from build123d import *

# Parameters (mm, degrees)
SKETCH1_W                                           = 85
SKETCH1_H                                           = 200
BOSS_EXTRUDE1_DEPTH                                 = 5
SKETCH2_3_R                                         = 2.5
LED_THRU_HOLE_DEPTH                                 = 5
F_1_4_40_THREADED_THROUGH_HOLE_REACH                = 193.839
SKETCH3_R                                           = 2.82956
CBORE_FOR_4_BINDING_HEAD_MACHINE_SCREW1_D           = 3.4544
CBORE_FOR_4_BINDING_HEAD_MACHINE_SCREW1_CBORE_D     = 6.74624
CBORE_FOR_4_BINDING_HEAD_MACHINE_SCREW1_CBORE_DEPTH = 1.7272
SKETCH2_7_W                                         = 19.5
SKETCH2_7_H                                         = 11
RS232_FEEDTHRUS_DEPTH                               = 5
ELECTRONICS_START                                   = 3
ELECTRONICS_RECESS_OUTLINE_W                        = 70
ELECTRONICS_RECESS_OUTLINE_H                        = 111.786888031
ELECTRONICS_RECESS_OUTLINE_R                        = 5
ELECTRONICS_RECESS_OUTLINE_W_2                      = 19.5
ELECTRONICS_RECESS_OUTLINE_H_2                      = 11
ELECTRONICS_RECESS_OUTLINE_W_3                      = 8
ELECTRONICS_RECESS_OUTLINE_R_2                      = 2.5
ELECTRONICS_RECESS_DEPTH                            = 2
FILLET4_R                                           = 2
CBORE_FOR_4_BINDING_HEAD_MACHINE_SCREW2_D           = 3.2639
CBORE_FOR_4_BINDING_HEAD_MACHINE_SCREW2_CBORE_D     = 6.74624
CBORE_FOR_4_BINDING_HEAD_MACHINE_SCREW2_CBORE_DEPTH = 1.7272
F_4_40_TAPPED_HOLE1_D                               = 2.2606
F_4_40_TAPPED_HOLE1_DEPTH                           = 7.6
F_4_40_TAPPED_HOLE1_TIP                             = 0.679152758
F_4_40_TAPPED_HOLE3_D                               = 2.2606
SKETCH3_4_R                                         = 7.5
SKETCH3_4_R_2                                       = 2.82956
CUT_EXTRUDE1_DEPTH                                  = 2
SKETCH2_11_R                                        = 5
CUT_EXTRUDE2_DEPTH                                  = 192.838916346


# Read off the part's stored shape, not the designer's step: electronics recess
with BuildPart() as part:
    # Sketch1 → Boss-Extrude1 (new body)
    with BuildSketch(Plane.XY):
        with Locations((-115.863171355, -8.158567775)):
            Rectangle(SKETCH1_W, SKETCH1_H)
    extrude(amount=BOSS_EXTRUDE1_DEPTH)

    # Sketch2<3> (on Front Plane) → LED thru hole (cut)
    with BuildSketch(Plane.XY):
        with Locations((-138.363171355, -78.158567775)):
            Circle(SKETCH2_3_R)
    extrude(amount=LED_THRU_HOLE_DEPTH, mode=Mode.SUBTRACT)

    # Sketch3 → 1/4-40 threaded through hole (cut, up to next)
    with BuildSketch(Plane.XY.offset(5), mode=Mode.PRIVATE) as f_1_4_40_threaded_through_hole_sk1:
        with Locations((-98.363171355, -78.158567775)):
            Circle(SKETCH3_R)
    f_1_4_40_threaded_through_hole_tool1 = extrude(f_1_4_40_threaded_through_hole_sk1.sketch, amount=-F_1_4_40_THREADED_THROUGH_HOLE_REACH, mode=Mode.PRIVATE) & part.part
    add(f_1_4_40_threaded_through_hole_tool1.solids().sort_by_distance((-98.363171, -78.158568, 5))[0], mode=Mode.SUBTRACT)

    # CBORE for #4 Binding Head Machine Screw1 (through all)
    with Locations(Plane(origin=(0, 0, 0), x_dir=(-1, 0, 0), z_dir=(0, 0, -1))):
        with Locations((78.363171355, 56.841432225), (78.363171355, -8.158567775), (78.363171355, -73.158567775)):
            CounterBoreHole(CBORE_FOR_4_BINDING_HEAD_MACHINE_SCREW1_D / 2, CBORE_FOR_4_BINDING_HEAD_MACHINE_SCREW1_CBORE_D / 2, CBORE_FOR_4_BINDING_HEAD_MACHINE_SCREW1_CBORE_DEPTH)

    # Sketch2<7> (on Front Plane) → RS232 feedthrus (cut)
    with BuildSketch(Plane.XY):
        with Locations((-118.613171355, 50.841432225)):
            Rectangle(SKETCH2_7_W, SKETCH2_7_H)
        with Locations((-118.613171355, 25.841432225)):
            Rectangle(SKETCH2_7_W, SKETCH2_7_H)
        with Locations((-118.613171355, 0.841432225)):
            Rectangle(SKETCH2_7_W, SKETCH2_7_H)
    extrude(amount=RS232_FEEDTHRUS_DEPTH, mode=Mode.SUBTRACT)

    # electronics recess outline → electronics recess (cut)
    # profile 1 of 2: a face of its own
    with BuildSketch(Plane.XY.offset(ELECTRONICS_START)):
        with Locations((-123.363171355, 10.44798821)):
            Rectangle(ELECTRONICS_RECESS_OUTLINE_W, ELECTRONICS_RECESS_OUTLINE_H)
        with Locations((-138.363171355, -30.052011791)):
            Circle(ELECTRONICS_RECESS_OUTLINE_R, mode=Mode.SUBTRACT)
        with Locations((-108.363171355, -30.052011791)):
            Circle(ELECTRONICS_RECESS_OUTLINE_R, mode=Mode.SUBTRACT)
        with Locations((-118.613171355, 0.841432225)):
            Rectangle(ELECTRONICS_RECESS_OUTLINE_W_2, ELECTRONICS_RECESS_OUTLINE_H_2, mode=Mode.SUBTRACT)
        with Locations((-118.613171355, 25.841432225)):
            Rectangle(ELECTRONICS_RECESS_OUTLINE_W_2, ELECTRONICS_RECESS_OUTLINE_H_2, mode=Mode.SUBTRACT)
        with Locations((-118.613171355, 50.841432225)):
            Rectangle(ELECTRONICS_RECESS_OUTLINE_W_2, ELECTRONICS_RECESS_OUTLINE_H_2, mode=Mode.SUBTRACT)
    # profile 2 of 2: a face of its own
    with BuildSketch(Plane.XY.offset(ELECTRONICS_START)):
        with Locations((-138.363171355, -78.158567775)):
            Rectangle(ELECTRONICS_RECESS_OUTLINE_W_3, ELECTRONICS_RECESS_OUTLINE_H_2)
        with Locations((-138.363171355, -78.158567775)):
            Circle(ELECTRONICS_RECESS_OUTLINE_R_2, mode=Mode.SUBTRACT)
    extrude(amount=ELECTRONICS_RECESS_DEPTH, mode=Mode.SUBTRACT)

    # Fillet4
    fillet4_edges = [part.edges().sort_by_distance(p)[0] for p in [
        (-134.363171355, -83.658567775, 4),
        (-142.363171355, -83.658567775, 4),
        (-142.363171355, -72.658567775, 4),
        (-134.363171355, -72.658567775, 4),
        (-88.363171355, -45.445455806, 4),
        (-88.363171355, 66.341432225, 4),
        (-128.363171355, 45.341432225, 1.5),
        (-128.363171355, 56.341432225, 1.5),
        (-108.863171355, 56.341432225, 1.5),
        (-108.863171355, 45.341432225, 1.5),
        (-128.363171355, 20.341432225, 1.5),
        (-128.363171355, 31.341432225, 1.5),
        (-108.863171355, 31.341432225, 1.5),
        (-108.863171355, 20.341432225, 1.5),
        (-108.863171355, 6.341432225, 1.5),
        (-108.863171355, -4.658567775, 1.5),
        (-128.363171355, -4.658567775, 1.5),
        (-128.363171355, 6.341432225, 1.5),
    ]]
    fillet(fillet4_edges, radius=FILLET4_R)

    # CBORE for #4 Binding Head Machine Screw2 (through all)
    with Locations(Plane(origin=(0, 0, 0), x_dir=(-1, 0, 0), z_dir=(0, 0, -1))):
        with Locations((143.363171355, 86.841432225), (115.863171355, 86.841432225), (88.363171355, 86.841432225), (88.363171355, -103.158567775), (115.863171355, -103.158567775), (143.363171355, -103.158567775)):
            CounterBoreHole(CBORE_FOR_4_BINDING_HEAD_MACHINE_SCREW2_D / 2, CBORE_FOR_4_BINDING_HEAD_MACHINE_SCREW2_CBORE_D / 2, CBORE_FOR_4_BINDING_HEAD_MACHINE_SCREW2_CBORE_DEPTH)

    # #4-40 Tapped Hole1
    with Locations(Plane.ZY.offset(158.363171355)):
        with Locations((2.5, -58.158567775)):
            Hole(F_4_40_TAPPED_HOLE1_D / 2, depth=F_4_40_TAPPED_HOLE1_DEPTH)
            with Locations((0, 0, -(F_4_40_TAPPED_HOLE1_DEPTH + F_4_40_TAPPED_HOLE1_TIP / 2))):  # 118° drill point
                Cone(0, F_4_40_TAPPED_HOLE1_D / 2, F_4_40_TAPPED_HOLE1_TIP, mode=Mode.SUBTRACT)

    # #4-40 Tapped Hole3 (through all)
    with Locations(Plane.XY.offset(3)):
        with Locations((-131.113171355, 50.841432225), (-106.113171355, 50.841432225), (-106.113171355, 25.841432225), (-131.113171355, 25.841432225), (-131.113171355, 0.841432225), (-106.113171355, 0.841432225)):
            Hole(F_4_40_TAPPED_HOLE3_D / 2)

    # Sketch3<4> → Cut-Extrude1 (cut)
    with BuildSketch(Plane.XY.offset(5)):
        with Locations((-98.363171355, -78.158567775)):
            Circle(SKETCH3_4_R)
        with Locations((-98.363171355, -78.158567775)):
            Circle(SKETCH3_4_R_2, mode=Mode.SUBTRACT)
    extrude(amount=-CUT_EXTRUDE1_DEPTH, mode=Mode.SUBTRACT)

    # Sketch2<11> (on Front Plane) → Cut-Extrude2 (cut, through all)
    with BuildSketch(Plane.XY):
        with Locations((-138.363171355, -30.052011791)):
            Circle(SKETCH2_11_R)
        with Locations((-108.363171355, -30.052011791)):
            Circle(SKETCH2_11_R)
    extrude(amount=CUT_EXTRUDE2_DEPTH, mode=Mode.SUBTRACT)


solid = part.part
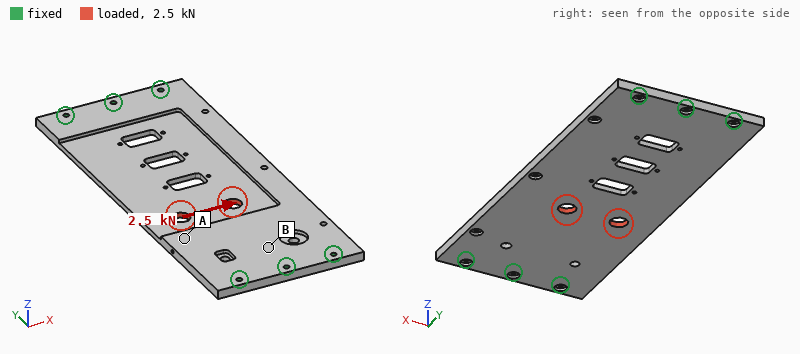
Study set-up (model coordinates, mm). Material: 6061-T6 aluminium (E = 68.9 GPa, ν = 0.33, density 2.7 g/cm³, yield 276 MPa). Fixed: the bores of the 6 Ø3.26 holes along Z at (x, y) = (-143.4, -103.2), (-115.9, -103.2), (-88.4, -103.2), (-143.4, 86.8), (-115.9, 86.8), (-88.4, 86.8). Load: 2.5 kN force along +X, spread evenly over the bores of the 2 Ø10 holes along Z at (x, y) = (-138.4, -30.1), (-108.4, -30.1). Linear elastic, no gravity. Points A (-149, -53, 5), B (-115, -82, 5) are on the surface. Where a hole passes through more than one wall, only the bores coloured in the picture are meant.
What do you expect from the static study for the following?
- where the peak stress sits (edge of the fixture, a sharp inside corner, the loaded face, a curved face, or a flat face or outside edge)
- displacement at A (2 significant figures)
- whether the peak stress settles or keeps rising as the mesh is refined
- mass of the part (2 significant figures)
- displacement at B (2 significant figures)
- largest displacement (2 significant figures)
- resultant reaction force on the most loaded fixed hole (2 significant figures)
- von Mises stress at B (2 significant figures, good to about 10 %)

edge of the fixture
33 µm
keeps rising
180 g
9.3 µm
55 µm
1.3 kN
11 MPa
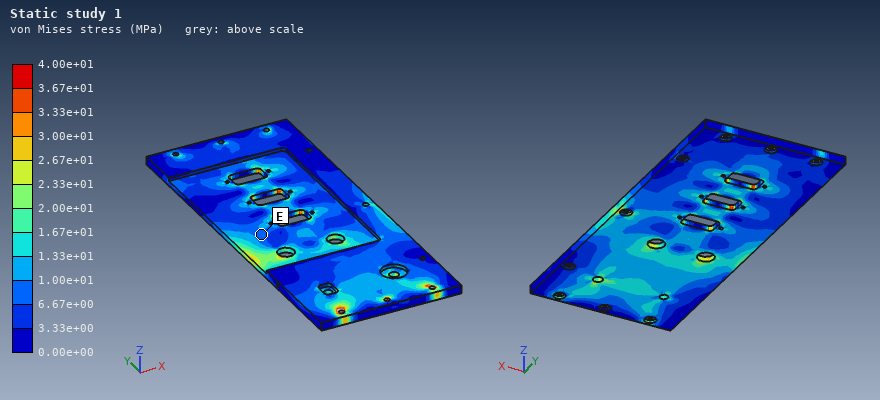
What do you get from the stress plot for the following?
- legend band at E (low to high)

6.67e+00 to 1.00e+01 MPa
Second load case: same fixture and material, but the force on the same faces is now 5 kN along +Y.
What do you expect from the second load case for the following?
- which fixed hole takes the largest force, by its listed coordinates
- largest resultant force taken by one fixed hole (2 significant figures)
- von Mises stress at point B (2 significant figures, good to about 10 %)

(-143.4, -103.2)
1.3 kN
8.7 MPa
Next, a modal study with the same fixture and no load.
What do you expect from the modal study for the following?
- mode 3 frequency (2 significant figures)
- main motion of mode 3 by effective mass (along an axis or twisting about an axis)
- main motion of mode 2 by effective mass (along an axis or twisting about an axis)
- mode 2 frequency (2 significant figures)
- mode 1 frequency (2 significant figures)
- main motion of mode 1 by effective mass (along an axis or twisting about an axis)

1500 Hz
twisting about X
twisting about Y
1000 Hz
610 Hz
along Z
